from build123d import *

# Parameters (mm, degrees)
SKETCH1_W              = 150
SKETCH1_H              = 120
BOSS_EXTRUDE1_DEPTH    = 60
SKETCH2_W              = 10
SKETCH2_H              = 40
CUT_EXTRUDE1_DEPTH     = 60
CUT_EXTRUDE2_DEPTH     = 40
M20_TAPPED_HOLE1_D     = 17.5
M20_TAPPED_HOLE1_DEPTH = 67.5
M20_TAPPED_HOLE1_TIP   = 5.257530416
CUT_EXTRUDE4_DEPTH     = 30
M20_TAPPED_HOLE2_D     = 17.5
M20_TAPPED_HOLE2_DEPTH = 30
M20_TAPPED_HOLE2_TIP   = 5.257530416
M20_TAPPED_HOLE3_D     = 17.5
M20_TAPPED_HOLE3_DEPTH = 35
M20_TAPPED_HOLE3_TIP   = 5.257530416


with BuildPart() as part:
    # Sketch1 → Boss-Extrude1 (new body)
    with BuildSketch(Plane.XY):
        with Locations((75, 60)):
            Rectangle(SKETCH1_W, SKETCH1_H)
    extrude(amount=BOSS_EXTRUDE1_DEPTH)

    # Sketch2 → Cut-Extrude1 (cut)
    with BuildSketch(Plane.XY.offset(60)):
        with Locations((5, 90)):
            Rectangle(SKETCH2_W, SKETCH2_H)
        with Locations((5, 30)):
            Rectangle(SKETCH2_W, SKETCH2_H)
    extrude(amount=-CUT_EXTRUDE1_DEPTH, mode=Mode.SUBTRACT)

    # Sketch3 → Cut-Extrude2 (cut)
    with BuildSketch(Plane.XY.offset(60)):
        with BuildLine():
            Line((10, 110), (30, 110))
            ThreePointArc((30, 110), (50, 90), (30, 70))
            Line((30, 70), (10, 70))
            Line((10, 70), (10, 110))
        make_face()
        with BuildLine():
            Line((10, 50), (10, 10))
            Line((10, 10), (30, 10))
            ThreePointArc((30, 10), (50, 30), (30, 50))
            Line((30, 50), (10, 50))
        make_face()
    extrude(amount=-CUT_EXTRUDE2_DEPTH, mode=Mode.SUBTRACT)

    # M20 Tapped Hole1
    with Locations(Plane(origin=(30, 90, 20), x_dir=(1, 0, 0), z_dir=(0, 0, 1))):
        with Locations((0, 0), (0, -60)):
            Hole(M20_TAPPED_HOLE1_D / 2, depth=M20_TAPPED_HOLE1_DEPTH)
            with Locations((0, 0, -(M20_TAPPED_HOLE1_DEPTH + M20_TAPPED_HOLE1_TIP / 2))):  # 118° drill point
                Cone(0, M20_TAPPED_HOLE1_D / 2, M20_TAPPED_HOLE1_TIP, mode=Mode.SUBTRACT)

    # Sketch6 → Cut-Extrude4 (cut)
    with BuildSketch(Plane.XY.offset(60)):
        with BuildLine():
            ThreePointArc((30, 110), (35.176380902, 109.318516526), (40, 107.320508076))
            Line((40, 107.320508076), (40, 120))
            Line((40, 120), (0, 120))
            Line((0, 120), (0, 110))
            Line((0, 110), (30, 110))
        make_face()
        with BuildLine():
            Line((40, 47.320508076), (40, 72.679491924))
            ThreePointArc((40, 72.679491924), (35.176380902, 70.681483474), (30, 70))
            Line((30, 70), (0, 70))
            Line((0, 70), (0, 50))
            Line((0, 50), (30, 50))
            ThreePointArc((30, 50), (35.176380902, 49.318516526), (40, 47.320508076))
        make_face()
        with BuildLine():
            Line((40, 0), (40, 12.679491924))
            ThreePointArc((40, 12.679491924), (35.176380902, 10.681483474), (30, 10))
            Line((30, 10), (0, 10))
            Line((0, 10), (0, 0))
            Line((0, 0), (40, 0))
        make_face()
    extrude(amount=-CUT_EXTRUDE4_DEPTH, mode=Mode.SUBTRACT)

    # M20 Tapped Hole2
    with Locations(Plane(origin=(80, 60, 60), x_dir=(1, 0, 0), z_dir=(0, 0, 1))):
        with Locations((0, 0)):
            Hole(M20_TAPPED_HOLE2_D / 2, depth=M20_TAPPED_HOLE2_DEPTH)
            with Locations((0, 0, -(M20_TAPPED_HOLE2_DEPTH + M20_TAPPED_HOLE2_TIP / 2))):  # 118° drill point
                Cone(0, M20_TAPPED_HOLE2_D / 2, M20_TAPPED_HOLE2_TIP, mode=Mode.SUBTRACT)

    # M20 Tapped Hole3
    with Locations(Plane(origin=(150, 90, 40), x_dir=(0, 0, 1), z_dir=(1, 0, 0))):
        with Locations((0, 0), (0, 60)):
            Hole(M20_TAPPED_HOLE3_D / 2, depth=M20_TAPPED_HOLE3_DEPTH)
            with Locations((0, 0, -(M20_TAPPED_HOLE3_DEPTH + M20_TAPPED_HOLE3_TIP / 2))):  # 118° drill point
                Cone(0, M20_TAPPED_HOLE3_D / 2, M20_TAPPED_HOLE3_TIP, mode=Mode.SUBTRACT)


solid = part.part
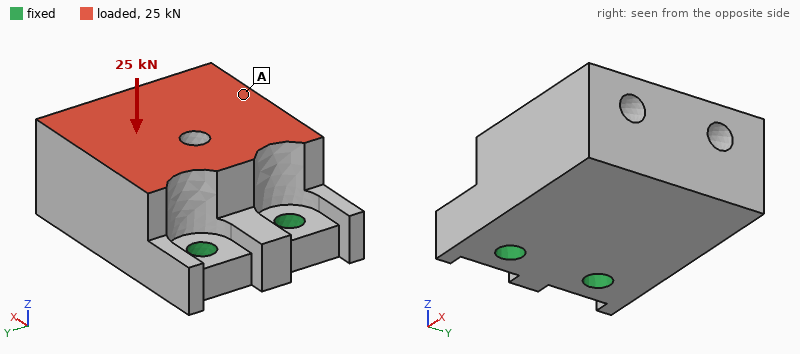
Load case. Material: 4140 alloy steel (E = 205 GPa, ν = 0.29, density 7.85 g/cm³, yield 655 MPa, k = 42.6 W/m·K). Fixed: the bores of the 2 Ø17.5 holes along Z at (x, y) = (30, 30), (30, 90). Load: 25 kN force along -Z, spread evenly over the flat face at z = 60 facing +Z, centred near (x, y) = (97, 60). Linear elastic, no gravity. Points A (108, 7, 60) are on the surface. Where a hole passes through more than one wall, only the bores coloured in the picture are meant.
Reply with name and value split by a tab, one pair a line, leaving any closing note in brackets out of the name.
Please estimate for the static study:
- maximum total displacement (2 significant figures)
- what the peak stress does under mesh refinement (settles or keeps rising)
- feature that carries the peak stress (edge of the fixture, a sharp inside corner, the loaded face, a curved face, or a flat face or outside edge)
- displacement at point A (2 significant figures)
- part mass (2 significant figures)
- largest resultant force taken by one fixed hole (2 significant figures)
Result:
maximum total displacement	0.17 mm
what the peak stress does under mesh refinement	keeps rising
feature that carries the peak stress	edge of the fixture
displacement at point A	0.12 mm
part mass	6.5 kg
largest resultant force taken by one fixed hole	13 kN
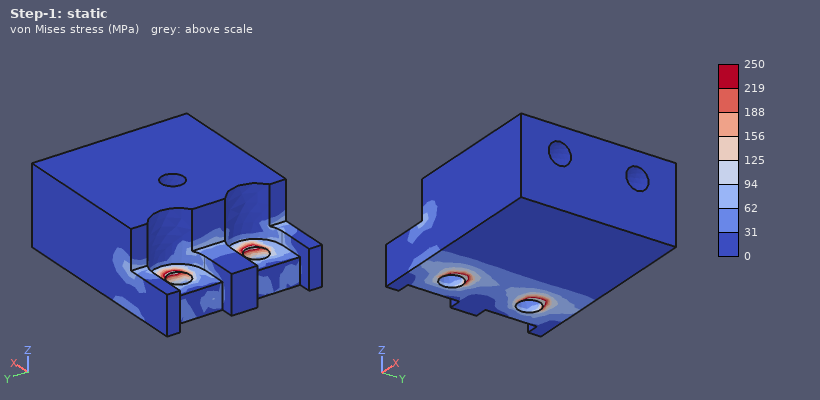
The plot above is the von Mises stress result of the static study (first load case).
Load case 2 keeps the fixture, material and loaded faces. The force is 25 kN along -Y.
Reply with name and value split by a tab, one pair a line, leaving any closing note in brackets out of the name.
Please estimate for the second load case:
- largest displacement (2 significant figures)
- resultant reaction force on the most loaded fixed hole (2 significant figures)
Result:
largest displacement	33 µm
resultant reaction force on the most loaded fixed hole	30 kN
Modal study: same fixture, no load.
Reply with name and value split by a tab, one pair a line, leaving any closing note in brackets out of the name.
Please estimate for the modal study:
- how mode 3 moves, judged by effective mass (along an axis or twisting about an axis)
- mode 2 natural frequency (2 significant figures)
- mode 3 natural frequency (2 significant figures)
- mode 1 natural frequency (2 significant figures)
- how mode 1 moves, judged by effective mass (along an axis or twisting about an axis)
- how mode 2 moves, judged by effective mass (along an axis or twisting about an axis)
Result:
how mode 3 moves, judged by effective mass	twisting about X
mode 2 natural frequency	2600 Hz
mode 3 natural frequency	3200 Hz
mode 1 natural frequency	970 Hz
how mode 1 moves, judged by effective mass	along Z
how mode 2 moves, judged by effective mass	along Y
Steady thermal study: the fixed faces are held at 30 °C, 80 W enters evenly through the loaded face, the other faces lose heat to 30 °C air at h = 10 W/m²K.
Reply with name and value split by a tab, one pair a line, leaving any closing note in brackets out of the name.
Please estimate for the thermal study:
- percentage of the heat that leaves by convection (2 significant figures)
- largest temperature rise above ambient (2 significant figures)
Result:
percentage of the heat that leaves by convection	13 %
largest temperature rise above ambient	31 K
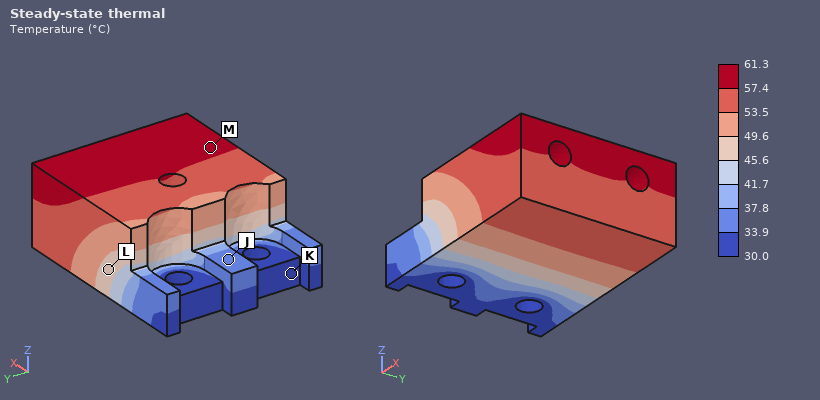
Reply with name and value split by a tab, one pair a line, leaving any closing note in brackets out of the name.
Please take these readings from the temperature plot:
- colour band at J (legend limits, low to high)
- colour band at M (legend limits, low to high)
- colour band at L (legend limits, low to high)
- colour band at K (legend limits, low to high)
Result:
colour band at J	33.9 to 37.8 °C
colour band at M	57.4 to 61.3 °C
colour band at L	45.6 to 49.6 °C
colour band at K	30.0 to 33.9 °C
